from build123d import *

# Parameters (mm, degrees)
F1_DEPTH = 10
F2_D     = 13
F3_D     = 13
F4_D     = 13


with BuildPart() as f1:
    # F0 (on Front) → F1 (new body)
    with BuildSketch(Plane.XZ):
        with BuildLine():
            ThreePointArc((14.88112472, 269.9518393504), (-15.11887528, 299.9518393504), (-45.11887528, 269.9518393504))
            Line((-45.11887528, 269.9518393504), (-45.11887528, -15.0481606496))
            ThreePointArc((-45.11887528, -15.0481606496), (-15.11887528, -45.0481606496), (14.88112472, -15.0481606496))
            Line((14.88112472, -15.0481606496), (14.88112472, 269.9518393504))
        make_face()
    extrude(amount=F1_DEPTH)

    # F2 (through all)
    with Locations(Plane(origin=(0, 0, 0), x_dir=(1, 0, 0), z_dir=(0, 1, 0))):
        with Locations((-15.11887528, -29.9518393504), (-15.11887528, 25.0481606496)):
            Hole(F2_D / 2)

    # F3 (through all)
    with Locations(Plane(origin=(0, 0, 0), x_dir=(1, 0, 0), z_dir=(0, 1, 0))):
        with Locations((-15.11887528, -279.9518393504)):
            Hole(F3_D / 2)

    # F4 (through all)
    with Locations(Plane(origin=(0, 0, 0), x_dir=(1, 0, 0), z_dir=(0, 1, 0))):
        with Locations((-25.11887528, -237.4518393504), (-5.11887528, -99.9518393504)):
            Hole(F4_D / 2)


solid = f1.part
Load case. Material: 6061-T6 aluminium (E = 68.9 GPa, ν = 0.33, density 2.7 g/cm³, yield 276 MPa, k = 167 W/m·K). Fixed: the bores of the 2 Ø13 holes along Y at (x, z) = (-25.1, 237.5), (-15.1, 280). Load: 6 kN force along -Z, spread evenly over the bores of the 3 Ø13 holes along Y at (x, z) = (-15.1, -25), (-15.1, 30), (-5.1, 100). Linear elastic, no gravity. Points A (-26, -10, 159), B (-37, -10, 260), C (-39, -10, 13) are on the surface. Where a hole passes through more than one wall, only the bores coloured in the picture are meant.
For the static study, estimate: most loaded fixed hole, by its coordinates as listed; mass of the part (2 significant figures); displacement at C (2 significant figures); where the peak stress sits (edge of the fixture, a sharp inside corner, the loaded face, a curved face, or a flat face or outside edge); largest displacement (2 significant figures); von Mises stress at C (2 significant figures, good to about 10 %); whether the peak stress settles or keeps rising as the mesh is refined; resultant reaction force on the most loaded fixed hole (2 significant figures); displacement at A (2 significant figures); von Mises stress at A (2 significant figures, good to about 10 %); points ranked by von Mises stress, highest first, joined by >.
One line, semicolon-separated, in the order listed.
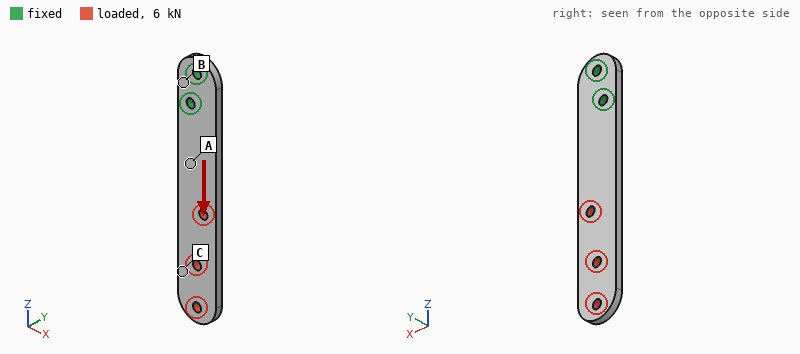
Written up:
(-25.1, 237.5); 520 g; 0.075 mm; edge of the fixture; 0.10 mm; 4.7 MPa; keeps rising; 4.3 kN; 0.020 mm; 8.8 MPa; A > C > B
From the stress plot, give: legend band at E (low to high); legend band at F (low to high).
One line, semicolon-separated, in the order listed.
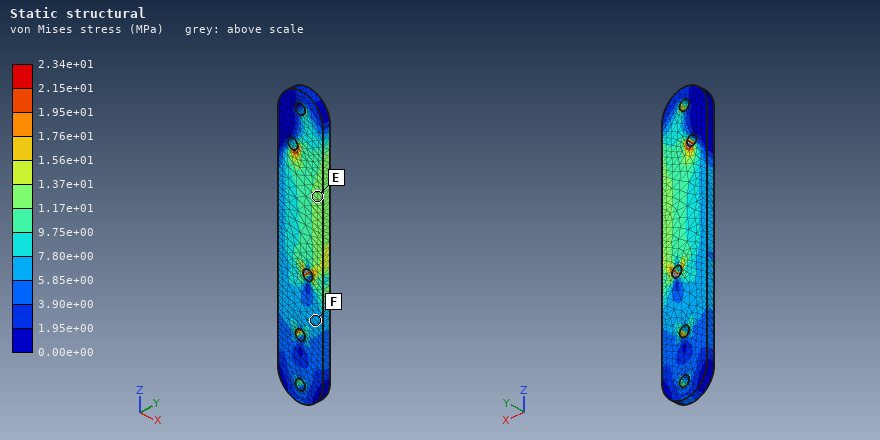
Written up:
1.17e+01 to 1.37e+01 MPa; 5.85e+00 to 7.80e+00 MPa
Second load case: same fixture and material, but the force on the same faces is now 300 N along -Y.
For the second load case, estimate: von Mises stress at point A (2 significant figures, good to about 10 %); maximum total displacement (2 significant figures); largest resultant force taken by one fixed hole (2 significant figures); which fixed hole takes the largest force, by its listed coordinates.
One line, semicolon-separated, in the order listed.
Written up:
37 MPa; 3.9 mm; 720 N; (-25.1, 237.5)
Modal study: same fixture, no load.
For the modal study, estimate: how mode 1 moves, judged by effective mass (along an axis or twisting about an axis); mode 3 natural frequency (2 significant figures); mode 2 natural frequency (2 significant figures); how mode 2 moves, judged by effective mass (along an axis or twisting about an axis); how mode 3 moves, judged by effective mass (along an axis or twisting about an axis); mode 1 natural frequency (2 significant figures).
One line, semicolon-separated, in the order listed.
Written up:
along Y; 670 Hz; 550 Hz; along X; along Y; 110 Hz
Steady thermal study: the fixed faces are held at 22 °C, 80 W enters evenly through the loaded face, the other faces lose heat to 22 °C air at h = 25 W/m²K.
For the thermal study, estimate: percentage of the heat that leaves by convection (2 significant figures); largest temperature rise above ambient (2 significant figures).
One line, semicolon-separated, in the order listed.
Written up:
58 %; 85 K
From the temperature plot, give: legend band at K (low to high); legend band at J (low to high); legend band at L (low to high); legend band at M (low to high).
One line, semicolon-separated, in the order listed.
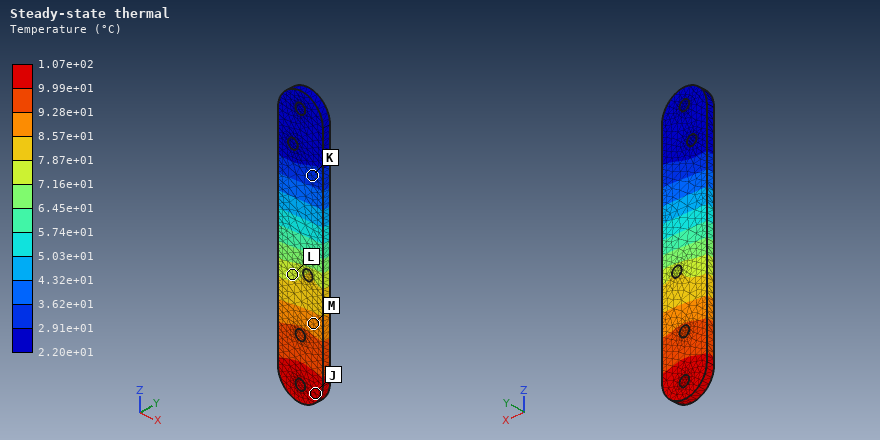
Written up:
2.91e+01 to 3.62e+01 °C; 9.99e+01 to 1.07e+02 °C; 7.16e+01 to 7.87e+01 °C; 8.57e+01 to 9.28e+01 °C
